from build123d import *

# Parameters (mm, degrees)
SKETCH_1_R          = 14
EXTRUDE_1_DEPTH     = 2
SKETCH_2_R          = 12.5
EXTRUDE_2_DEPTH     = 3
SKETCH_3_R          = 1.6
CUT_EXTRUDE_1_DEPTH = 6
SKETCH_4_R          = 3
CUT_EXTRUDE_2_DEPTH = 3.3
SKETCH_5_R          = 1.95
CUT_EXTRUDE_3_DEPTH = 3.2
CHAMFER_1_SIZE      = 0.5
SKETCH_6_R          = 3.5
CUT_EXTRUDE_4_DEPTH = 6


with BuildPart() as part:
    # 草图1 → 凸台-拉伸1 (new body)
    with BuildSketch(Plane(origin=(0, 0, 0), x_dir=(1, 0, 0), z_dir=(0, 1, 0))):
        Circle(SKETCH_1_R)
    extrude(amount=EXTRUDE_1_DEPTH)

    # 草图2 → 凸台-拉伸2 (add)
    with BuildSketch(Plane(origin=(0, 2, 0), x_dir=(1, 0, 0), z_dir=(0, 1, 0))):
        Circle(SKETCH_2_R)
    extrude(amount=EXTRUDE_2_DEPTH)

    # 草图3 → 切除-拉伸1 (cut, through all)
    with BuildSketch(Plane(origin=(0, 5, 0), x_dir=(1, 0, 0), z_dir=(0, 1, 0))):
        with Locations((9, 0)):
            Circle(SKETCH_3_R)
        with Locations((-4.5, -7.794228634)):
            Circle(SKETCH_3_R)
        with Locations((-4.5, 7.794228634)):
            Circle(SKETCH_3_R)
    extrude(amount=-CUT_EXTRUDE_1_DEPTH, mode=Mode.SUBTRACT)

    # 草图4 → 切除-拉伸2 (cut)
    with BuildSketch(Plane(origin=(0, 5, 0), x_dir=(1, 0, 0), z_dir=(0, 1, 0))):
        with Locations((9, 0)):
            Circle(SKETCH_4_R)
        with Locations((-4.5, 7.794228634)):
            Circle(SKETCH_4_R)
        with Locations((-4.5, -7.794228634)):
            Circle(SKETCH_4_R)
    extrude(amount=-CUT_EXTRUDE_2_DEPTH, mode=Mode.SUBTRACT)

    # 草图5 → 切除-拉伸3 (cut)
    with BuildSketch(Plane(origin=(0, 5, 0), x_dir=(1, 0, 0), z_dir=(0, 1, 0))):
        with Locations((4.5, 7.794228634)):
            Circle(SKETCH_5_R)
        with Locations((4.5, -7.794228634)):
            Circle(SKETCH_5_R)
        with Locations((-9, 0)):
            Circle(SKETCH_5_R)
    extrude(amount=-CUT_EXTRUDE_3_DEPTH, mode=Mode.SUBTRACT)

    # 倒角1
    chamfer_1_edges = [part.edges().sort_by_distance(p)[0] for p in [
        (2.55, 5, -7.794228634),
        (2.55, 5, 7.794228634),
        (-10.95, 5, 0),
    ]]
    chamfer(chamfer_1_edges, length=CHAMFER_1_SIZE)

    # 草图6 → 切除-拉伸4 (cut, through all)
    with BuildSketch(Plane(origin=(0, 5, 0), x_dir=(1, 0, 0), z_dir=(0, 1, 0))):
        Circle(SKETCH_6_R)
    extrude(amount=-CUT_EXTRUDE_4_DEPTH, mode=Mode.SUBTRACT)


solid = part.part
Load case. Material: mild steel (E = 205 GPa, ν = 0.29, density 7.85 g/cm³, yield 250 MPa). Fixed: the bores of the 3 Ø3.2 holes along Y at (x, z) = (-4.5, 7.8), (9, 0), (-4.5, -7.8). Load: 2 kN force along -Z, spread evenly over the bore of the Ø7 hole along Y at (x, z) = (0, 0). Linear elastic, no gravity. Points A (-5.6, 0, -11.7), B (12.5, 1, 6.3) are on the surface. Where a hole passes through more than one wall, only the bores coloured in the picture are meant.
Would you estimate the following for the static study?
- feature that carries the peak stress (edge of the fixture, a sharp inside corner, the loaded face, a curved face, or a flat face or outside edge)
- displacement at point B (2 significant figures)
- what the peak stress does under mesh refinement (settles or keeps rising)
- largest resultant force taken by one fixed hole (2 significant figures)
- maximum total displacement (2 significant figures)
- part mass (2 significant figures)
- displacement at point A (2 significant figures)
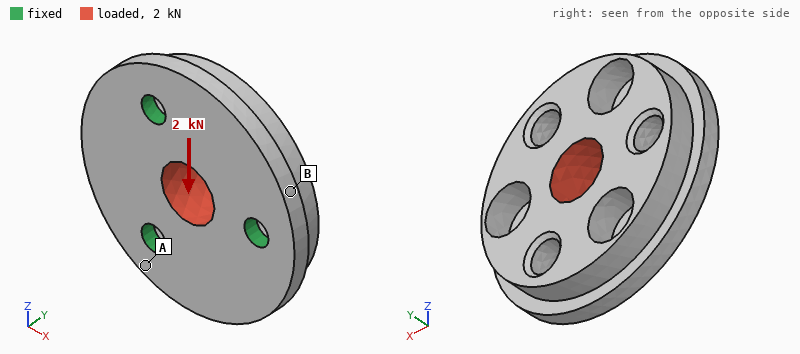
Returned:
edge of the fixture
1.5 µm
keeps rising
720 N
2.6 µm
16 g
0.52 µm
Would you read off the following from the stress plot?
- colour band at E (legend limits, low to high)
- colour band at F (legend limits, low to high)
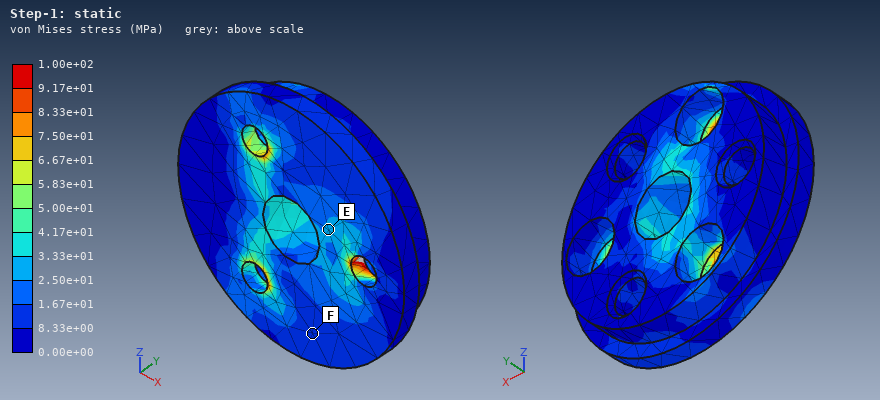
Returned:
2.50e+01 to 3.33e+01 MPa
8.33e+00 to 1.67e+01 MPa
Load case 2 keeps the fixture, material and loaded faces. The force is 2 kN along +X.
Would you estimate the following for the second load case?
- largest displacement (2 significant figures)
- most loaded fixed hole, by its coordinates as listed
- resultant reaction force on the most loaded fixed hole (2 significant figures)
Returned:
2.9 µm
(9, 0)
750 N
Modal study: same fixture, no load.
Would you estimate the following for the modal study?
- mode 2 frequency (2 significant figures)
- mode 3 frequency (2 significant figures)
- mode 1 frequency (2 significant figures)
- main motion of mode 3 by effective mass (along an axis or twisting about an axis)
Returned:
26 kHz
35 kHz
26 kHz
along Y
